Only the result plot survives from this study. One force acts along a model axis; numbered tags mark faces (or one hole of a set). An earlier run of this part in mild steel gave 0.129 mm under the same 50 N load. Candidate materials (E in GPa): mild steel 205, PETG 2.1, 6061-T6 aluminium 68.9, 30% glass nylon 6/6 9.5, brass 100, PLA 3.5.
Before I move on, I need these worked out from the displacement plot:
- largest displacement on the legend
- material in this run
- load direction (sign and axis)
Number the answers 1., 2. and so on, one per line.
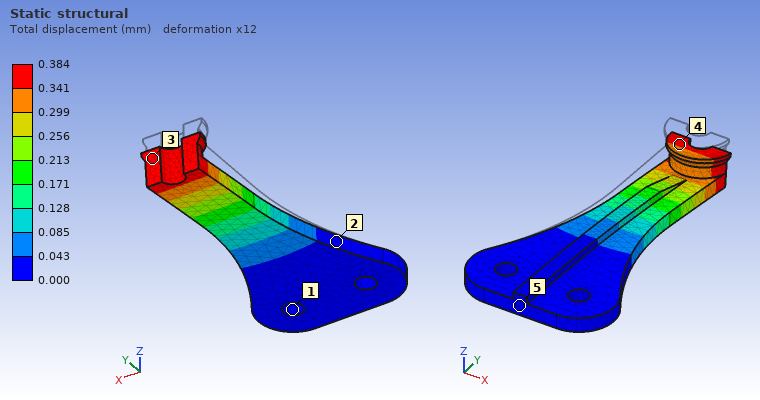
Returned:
1. 0.384 mm
2. 6061-T6 aluminium
3. -Z
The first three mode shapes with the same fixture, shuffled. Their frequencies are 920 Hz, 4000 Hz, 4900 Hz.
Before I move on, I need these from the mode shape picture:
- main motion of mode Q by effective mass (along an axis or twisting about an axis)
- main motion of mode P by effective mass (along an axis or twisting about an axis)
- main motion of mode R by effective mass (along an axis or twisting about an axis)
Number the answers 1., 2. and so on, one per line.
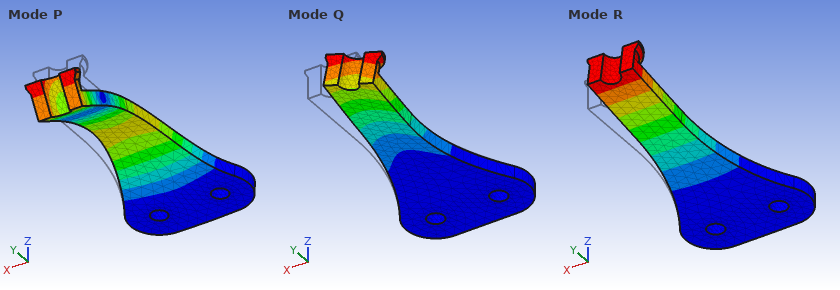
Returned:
1. along X
2. along Z
3. along Z
